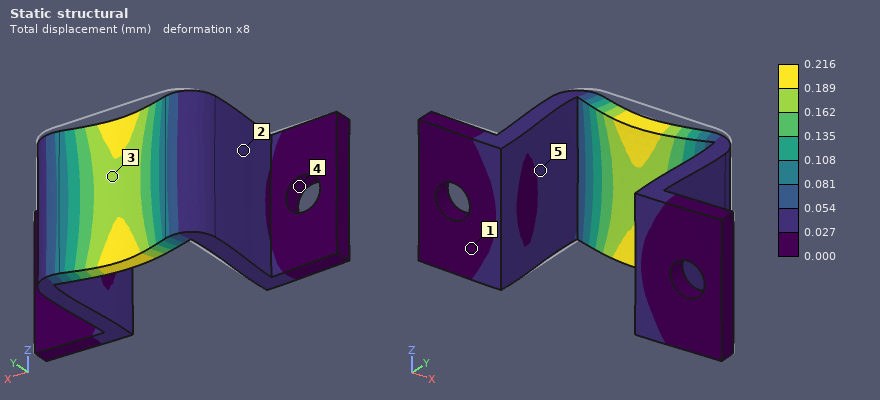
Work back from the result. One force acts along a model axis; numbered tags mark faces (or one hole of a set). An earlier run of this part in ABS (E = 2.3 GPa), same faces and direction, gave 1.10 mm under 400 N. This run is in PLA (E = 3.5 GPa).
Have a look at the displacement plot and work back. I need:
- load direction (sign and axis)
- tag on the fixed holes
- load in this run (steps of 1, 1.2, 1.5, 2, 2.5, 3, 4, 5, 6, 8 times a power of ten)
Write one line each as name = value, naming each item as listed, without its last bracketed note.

load direction = -Y
tag on the fixed holes = 4
load in this run = 120 N
